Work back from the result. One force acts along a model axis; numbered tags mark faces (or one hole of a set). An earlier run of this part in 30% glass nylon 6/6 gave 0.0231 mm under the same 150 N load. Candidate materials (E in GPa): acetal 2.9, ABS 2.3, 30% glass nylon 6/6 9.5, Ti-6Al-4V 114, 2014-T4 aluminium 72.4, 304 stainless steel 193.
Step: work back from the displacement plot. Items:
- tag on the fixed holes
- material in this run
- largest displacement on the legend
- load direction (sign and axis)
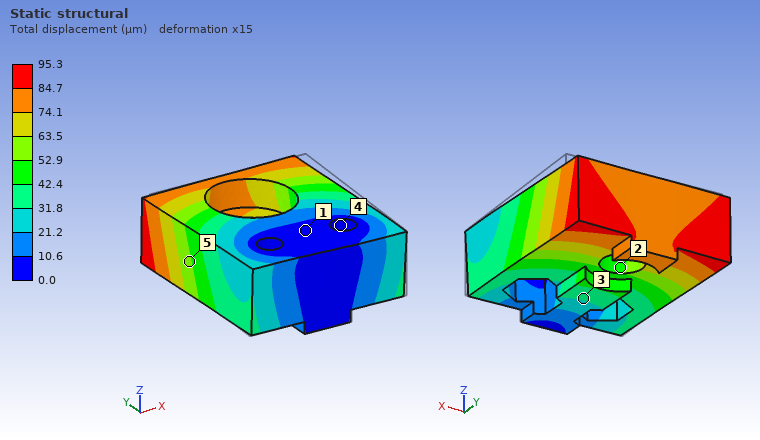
4
ABS
95.3 µm
-X
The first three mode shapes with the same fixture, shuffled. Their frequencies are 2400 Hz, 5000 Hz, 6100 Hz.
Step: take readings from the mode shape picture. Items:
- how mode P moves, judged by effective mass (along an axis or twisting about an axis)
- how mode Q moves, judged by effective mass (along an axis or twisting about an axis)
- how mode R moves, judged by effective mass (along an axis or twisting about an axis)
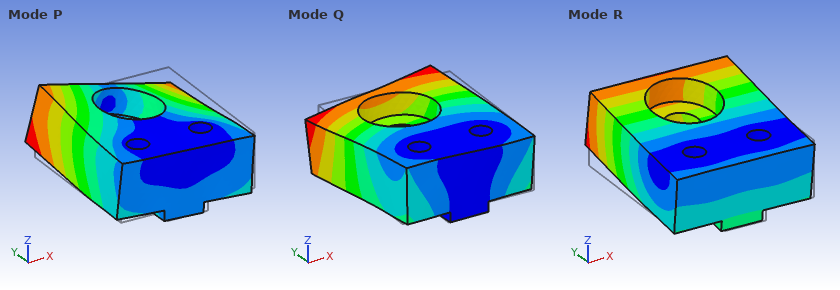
along X
along X
along Z
